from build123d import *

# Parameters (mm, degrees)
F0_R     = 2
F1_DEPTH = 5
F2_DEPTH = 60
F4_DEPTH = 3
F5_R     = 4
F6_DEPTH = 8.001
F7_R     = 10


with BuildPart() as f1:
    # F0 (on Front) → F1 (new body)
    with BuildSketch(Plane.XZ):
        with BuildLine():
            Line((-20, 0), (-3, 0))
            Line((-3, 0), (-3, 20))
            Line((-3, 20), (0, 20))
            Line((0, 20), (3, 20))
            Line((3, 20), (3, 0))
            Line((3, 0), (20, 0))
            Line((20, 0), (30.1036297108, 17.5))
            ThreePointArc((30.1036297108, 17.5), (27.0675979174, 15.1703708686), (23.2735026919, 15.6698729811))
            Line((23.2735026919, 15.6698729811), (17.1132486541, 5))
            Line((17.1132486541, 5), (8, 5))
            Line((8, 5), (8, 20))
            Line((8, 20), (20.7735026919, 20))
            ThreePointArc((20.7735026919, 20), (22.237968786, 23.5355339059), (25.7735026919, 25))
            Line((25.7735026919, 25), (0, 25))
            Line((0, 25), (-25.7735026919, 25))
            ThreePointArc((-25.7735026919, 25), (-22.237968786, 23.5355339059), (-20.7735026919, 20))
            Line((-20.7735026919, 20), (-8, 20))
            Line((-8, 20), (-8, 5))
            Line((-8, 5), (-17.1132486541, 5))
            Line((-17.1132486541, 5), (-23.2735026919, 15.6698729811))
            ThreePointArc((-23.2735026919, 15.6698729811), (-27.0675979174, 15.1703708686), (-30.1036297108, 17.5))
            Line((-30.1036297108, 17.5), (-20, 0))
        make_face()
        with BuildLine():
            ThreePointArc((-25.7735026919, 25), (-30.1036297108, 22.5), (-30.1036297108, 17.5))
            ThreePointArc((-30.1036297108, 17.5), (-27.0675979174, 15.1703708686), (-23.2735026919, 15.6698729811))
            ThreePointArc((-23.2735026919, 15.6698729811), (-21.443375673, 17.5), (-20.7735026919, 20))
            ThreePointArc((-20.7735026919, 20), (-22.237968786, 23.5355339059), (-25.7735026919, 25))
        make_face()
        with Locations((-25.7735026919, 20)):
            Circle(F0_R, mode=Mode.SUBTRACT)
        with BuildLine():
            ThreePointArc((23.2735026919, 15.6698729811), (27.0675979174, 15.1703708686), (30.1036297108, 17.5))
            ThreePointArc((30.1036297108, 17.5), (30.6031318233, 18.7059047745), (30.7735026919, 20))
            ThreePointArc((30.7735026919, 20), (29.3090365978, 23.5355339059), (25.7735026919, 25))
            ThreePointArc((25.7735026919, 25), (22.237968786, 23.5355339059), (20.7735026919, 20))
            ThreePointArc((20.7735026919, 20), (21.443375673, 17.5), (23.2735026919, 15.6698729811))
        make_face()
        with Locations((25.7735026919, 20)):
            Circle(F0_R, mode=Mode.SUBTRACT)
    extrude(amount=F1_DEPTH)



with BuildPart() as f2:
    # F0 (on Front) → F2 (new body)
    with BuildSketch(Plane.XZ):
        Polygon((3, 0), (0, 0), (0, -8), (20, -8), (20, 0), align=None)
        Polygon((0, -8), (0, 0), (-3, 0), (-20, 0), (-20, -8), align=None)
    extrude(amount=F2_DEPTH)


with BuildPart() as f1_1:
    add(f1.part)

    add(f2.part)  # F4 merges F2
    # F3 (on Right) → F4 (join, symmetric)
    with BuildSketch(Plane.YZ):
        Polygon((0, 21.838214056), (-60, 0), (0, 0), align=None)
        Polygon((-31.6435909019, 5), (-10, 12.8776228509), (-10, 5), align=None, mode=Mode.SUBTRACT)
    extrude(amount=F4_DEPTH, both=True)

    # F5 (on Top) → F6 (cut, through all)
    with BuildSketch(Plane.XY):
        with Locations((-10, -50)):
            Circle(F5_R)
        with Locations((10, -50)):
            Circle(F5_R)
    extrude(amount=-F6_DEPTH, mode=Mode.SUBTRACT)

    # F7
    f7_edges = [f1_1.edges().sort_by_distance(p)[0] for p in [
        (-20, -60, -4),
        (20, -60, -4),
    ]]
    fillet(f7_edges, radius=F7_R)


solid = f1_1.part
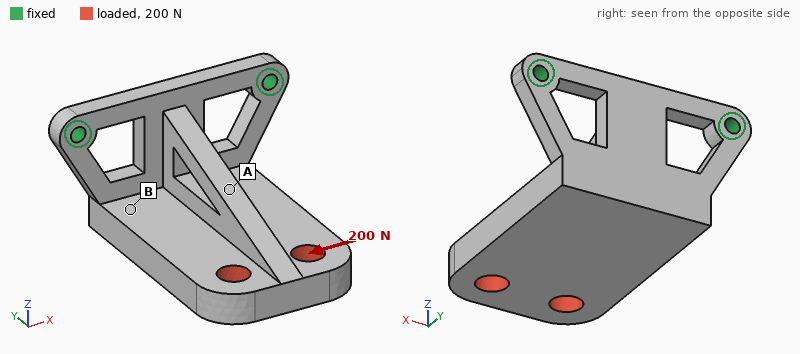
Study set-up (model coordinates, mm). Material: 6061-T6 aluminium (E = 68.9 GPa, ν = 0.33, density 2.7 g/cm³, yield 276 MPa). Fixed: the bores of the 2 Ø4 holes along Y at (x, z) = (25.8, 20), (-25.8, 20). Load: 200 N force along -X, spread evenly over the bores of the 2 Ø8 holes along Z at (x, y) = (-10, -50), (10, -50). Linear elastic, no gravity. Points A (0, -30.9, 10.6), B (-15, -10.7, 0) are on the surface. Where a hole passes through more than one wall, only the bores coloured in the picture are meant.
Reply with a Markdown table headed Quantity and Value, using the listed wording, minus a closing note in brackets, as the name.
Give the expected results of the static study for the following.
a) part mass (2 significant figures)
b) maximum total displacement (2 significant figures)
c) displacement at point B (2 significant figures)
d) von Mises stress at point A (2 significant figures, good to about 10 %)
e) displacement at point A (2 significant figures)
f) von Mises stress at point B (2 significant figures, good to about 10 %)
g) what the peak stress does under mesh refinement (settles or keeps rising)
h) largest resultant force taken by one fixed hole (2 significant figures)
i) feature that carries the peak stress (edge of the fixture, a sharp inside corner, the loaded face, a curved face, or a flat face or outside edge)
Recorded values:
| Quantity | Value |
|---|---|
| part mass | 69 g |
| maximum total displacement | 0.12 mm |
| displacement at point B | 0.035 mm |
| von Mises stress at point A | 5.4 MPa |
| displacement at point A | 0.060 mm |
| von Mises stress at point B | 10 MPa |
| what the peak stress does under mesh refinement | keeps rising |
| largest resultant force taken by one fixed hole | 260 N |
| feature that carries the peak stress | edge of the fixture |
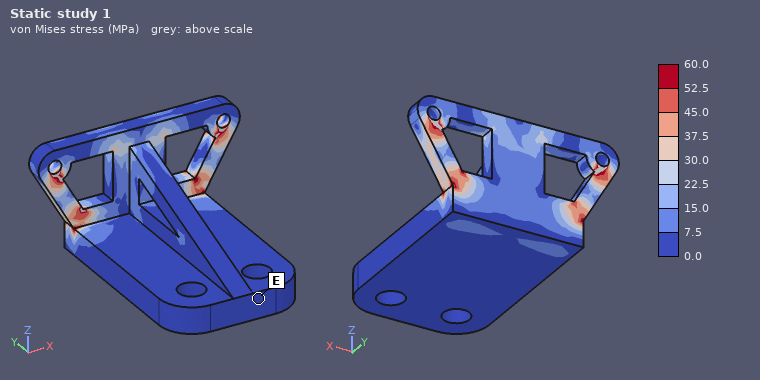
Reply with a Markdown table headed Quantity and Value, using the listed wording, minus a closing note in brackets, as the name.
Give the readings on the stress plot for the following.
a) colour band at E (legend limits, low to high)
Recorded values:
| Quantity | Value |
|---|---|
| colour band at E | 0.0 to 7.5 MPa |
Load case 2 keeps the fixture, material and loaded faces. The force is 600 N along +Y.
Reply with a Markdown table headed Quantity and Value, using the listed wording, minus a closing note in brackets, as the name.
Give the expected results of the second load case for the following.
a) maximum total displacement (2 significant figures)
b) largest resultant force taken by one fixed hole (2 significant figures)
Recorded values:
| Quantity | Value |
|---|---|
| maximum total displacement | 0.60 mm |
| largest resultant force taken by one fixed hole | 300 N |
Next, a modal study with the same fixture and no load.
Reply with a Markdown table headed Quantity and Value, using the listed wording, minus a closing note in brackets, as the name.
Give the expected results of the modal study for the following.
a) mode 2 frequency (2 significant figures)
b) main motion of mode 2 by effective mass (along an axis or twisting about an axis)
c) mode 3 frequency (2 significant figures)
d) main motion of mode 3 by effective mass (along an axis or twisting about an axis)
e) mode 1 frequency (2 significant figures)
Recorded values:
| Quantity | Value |
|---|---|
| mode 2 frequency | 1400 Hz |
| main motion of mode 2 by effective mass | along X |
| mode 3 frequency | 2700 Hz |
| main motion of mode 3 by effective mass | along Y |
| mode 1 frequency | 640 Hz |
